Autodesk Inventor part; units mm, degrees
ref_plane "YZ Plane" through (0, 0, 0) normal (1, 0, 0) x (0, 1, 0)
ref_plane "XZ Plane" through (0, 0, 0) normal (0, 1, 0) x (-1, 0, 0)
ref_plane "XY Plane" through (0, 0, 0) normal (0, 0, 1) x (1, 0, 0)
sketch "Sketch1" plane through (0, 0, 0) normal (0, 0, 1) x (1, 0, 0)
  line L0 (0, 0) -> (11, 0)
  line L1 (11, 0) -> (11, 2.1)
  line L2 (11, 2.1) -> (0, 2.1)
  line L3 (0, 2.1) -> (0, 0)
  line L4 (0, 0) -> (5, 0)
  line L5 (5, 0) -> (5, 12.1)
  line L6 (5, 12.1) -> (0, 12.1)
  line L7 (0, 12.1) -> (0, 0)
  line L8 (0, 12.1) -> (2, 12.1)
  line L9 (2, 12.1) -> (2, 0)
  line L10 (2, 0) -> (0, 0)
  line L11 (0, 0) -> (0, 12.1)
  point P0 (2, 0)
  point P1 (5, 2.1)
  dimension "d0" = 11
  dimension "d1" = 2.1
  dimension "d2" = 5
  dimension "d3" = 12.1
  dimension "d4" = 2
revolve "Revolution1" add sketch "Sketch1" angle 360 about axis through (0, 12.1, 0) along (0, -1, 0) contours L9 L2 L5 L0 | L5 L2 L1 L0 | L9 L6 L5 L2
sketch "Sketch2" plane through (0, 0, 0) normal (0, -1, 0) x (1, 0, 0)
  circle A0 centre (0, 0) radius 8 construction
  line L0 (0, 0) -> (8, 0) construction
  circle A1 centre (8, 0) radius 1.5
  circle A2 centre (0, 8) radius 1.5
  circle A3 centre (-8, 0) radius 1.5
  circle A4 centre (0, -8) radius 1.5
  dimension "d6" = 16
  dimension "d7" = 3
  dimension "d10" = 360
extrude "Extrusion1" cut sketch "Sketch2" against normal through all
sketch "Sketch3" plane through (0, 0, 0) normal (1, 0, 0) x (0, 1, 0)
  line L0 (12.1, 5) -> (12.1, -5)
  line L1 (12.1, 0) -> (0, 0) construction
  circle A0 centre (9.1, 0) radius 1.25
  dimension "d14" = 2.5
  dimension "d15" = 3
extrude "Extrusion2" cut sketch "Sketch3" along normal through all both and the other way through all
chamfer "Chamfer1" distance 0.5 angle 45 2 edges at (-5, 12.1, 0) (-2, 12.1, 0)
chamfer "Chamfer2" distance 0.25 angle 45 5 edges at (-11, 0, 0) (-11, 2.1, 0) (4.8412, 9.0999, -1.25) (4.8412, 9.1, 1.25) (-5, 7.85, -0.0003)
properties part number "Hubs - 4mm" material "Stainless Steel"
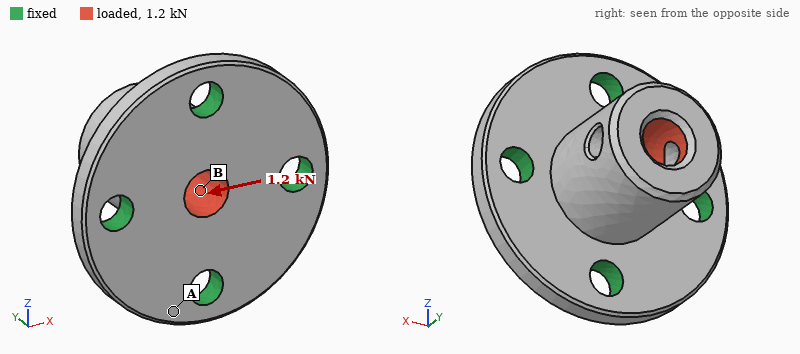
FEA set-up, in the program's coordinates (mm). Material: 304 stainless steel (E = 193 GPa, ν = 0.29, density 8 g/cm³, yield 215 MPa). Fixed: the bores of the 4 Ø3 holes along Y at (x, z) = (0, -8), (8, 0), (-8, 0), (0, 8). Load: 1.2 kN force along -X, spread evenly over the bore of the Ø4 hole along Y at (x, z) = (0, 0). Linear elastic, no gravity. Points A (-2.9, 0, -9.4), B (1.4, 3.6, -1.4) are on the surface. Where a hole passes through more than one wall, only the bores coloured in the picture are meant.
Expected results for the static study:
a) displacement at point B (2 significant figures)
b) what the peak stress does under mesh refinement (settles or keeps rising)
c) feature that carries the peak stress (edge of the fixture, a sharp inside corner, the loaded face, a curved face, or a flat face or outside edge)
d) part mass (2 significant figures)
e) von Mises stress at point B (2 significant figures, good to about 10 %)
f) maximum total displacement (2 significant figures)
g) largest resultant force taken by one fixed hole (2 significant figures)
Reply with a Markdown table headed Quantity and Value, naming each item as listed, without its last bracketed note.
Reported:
| Quantity | Value |
|---|---|
| displacement at point B | 1.8 µm |
| what the peak stress does under mesh refinement | keeps rising |
| feature that carries the peak stress | edge of the fixture |
| part mass | 11 g |
| von Mises stress at point B | 28 MPa |
| maximum total displacement | 7.2 µm |
| largest resultant force taken by one fixed hole | 580 N |
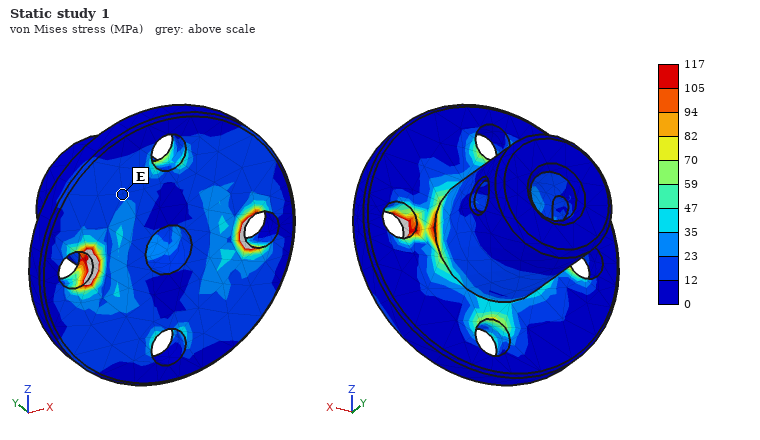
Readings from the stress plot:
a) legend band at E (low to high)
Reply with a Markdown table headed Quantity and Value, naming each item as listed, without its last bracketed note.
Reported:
| Quantity | Value |
|---|---|
| legend band at E | 12 to 23 MPa |
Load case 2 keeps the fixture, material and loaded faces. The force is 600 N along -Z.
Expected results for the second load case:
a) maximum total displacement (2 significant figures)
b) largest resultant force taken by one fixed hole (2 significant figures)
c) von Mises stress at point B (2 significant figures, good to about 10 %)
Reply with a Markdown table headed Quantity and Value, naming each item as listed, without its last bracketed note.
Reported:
| Quantity | Value |
|---|---|
| maximum total displacement | 3.7 µm |
| largest resultant force taken by one fixed hole | 290 N |
| von Mises stress at point B | 14 MPa |
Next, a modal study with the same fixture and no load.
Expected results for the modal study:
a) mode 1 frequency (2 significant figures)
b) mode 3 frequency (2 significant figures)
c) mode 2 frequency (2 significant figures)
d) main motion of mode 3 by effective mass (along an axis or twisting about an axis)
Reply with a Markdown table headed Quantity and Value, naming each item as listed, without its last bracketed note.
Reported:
| Quantity | Value |
|---|---|
| mode 1 frequency | 29 kHz |
| mode 3 frequency | 49 kHz |
| mode 2 frequency | 30 kHz |
| main motion of mode 3 by effective mass | along Y |
